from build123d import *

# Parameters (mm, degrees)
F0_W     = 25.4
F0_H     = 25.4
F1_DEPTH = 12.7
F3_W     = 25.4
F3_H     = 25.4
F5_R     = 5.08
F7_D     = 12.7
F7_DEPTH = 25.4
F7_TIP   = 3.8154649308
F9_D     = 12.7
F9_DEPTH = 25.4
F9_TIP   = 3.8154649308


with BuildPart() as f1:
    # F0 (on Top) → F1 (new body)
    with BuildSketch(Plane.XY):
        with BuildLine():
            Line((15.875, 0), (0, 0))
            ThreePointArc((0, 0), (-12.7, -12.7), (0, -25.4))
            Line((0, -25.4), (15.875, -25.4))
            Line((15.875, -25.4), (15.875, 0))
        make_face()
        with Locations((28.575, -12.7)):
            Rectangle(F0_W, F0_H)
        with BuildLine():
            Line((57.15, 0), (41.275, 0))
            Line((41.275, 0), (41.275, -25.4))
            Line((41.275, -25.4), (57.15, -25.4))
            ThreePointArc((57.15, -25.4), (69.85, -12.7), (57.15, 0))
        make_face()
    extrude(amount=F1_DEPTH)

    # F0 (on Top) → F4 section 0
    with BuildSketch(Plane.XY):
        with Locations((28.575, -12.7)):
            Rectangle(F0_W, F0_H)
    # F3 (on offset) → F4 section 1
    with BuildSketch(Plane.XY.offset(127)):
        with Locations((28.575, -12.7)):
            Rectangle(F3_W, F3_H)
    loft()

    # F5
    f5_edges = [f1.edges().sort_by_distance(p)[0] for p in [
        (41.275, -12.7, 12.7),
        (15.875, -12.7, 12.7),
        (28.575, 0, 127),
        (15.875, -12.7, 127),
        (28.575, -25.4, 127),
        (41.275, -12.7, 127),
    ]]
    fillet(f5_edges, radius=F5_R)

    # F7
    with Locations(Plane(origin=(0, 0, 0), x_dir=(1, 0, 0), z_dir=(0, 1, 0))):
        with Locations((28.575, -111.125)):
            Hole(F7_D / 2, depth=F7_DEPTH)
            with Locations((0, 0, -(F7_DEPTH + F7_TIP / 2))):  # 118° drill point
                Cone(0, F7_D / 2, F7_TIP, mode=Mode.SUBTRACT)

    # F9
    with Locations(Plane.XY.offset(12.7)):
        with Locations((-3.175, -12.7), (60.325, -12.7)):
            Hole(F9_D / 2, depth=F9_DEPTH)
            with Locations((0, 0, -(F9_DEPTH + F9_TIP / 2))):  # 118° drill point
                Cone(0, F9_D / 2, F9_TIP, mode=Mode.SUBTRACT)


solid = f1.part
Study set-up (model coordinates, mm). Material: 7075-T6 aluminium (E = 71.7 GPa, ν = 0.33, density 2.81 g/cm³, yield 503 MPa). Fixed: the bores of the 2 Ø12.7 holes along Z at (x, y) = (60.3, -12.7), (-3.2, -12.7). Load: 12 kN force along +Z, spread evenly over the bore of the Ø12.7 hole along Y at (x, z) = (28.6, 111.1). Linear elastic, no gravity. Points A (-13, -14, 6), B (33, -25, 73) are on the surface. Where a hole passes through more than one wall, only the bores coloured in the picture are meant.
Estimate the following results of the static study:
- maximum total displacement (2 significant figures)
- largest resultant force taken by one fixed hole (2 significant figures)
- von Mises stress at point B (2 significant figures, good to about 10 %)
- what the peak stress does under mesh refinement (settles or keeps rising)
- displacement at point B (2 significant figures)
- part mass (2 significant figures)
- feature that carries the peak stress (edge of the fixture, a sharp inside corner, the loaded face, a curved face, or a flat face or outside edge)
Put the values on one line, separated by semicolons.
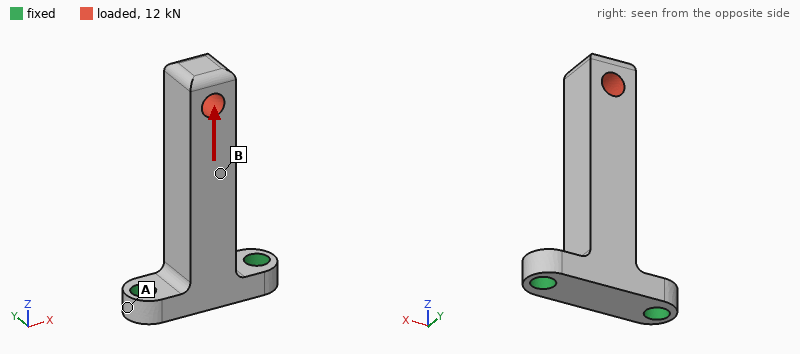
55 µm; 6.4 kN; 19 MPa; keeps rising; 39 µm; 260 g; edge of the fixture
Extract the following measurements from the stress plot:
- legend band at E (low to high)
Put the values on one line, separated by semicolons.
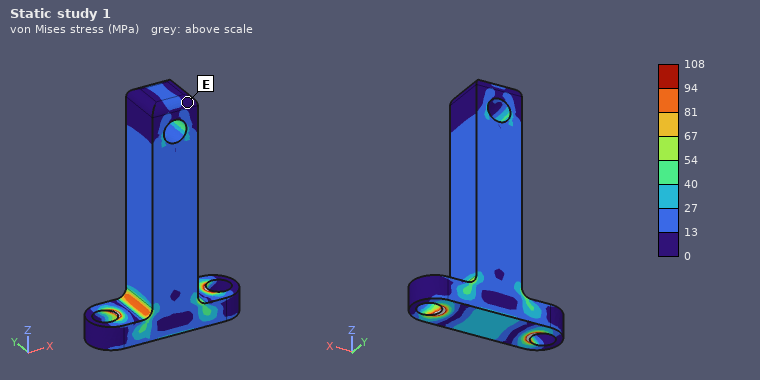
0 to 13 MPa
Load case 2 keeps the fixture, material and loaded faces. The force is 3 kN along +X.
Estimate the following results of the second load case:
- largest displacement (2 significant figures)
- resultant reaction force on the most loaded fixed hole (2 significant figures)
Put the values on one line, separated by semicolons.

0.67 mm; 7.3 kN
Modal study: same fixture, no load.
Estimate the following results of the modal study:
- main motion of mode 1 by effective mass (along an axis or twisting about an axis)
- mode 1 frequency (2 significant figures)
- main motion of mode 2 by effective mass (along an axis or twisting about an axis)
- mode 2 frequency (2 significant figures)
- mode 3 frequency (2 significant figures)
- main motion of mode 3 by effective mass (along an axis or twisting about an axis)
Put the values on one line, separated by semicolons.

along Y; 910 Hz; along X; 1400 Hz; 6000 Hz; along Y
